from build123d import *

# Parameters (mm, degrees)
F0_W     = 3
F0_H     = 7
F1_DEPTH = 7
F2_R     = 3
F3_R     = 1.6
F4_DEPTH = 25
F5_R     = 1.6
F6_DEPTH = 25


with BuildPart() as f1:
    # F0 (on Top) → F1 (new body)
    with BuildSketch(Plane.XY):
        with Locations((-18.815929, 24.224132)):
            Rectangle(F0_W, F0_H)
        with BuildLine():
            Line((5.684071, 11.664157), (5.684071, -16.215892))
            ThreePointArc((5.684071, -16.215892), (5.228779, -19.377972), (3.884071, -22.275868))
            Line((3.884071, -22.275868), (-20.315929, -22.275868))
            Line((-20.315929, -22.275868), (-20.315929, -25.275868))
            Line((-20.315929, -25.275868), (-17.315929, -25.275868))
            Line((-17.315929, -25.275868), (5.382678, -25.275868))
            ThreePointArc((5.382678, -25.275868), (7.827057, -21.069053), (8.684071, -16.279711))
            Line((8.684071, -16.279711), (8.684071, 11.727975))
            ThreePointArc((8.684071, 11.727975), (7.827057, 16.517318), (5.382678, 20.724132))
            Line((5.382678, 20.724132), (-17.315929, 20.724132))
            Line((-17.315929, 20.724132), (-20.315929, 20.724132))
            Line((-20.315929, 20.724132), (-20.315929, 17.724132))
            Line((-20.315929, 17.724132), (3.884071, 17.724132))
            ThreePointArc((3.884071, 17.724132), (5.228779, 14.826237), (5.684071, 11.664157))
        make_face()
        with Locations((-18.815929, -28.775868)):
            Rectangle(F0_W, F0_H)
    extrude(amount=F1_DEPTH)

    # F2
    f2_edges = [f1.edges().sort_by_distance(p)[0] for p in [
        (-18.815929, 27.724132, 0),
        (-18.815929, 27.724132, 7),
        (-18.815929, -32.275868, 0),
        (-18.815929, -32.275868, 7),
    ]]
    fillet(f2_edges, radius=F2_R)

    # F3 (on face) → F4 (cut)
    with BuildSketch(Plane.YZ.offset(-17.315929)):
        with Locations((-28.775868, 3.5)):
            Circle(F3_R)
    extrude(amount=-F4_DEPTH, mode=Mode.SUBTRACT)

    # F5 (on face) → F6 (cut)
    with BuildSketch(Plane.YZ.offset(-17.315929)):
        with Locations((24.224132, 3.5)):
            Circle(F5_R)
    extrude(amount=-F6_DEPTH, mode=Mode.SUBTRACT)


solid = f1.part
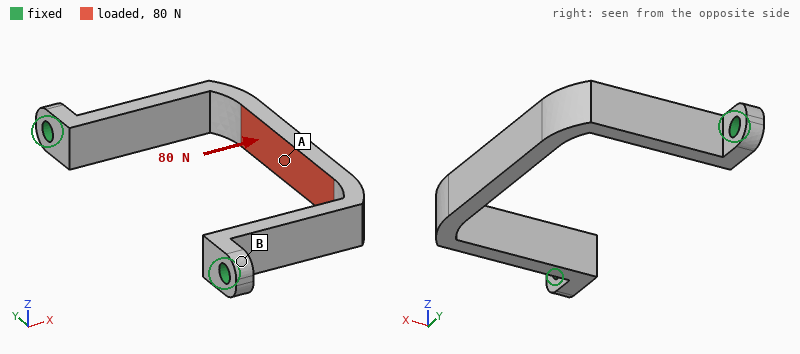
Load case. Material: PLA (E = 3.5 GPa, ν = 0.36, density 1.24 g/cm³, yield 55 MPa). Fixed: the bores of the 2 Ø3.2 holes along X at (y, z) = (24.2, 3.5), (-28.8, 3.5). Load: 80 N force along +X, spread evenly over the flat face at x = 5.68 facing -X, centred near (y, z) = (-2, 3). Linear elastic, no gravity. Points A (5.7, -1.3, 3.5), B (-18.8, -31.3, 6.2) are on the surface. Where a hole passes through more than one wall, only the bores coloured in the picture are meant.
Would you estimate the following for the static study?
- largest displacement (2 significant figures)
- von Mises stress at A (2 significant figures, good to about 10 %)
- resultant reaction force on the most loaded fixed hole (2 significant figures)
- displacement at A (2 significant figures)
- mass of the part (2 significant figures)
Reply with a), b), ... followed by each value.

a) 0.70 mm
b) 24 MPa
c) 44 N
d) 0.69 mm
e) 2.7 g
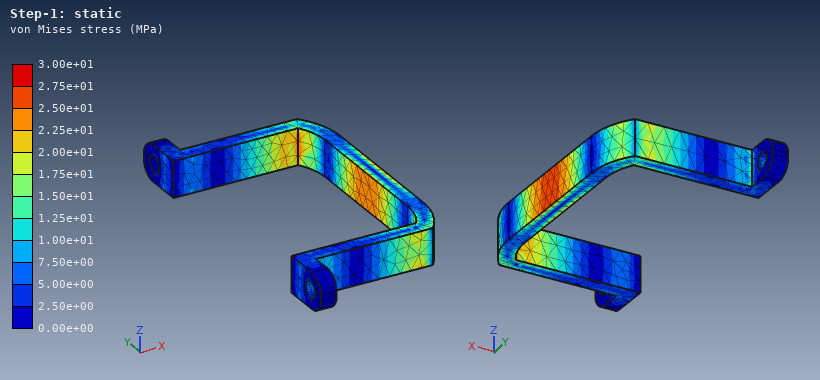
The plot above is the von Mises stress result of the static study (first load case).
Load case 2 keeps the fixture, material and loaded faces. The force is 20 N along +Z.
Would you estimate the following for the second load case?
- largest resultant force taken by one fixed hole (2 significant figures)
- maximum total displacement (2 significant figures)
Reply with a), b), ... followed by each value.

a) 10 N
b) 0.56 mm
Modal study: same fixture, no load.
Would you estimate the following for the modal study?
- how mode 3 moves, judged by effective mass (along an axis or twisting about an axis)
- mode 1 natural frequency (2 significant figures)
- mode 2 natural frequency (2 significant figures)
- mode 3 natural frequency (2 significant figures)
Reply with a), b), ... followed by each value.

a) twisting about X
b) 840 Hz
c) 850 Hz
d) 1500 Hz
